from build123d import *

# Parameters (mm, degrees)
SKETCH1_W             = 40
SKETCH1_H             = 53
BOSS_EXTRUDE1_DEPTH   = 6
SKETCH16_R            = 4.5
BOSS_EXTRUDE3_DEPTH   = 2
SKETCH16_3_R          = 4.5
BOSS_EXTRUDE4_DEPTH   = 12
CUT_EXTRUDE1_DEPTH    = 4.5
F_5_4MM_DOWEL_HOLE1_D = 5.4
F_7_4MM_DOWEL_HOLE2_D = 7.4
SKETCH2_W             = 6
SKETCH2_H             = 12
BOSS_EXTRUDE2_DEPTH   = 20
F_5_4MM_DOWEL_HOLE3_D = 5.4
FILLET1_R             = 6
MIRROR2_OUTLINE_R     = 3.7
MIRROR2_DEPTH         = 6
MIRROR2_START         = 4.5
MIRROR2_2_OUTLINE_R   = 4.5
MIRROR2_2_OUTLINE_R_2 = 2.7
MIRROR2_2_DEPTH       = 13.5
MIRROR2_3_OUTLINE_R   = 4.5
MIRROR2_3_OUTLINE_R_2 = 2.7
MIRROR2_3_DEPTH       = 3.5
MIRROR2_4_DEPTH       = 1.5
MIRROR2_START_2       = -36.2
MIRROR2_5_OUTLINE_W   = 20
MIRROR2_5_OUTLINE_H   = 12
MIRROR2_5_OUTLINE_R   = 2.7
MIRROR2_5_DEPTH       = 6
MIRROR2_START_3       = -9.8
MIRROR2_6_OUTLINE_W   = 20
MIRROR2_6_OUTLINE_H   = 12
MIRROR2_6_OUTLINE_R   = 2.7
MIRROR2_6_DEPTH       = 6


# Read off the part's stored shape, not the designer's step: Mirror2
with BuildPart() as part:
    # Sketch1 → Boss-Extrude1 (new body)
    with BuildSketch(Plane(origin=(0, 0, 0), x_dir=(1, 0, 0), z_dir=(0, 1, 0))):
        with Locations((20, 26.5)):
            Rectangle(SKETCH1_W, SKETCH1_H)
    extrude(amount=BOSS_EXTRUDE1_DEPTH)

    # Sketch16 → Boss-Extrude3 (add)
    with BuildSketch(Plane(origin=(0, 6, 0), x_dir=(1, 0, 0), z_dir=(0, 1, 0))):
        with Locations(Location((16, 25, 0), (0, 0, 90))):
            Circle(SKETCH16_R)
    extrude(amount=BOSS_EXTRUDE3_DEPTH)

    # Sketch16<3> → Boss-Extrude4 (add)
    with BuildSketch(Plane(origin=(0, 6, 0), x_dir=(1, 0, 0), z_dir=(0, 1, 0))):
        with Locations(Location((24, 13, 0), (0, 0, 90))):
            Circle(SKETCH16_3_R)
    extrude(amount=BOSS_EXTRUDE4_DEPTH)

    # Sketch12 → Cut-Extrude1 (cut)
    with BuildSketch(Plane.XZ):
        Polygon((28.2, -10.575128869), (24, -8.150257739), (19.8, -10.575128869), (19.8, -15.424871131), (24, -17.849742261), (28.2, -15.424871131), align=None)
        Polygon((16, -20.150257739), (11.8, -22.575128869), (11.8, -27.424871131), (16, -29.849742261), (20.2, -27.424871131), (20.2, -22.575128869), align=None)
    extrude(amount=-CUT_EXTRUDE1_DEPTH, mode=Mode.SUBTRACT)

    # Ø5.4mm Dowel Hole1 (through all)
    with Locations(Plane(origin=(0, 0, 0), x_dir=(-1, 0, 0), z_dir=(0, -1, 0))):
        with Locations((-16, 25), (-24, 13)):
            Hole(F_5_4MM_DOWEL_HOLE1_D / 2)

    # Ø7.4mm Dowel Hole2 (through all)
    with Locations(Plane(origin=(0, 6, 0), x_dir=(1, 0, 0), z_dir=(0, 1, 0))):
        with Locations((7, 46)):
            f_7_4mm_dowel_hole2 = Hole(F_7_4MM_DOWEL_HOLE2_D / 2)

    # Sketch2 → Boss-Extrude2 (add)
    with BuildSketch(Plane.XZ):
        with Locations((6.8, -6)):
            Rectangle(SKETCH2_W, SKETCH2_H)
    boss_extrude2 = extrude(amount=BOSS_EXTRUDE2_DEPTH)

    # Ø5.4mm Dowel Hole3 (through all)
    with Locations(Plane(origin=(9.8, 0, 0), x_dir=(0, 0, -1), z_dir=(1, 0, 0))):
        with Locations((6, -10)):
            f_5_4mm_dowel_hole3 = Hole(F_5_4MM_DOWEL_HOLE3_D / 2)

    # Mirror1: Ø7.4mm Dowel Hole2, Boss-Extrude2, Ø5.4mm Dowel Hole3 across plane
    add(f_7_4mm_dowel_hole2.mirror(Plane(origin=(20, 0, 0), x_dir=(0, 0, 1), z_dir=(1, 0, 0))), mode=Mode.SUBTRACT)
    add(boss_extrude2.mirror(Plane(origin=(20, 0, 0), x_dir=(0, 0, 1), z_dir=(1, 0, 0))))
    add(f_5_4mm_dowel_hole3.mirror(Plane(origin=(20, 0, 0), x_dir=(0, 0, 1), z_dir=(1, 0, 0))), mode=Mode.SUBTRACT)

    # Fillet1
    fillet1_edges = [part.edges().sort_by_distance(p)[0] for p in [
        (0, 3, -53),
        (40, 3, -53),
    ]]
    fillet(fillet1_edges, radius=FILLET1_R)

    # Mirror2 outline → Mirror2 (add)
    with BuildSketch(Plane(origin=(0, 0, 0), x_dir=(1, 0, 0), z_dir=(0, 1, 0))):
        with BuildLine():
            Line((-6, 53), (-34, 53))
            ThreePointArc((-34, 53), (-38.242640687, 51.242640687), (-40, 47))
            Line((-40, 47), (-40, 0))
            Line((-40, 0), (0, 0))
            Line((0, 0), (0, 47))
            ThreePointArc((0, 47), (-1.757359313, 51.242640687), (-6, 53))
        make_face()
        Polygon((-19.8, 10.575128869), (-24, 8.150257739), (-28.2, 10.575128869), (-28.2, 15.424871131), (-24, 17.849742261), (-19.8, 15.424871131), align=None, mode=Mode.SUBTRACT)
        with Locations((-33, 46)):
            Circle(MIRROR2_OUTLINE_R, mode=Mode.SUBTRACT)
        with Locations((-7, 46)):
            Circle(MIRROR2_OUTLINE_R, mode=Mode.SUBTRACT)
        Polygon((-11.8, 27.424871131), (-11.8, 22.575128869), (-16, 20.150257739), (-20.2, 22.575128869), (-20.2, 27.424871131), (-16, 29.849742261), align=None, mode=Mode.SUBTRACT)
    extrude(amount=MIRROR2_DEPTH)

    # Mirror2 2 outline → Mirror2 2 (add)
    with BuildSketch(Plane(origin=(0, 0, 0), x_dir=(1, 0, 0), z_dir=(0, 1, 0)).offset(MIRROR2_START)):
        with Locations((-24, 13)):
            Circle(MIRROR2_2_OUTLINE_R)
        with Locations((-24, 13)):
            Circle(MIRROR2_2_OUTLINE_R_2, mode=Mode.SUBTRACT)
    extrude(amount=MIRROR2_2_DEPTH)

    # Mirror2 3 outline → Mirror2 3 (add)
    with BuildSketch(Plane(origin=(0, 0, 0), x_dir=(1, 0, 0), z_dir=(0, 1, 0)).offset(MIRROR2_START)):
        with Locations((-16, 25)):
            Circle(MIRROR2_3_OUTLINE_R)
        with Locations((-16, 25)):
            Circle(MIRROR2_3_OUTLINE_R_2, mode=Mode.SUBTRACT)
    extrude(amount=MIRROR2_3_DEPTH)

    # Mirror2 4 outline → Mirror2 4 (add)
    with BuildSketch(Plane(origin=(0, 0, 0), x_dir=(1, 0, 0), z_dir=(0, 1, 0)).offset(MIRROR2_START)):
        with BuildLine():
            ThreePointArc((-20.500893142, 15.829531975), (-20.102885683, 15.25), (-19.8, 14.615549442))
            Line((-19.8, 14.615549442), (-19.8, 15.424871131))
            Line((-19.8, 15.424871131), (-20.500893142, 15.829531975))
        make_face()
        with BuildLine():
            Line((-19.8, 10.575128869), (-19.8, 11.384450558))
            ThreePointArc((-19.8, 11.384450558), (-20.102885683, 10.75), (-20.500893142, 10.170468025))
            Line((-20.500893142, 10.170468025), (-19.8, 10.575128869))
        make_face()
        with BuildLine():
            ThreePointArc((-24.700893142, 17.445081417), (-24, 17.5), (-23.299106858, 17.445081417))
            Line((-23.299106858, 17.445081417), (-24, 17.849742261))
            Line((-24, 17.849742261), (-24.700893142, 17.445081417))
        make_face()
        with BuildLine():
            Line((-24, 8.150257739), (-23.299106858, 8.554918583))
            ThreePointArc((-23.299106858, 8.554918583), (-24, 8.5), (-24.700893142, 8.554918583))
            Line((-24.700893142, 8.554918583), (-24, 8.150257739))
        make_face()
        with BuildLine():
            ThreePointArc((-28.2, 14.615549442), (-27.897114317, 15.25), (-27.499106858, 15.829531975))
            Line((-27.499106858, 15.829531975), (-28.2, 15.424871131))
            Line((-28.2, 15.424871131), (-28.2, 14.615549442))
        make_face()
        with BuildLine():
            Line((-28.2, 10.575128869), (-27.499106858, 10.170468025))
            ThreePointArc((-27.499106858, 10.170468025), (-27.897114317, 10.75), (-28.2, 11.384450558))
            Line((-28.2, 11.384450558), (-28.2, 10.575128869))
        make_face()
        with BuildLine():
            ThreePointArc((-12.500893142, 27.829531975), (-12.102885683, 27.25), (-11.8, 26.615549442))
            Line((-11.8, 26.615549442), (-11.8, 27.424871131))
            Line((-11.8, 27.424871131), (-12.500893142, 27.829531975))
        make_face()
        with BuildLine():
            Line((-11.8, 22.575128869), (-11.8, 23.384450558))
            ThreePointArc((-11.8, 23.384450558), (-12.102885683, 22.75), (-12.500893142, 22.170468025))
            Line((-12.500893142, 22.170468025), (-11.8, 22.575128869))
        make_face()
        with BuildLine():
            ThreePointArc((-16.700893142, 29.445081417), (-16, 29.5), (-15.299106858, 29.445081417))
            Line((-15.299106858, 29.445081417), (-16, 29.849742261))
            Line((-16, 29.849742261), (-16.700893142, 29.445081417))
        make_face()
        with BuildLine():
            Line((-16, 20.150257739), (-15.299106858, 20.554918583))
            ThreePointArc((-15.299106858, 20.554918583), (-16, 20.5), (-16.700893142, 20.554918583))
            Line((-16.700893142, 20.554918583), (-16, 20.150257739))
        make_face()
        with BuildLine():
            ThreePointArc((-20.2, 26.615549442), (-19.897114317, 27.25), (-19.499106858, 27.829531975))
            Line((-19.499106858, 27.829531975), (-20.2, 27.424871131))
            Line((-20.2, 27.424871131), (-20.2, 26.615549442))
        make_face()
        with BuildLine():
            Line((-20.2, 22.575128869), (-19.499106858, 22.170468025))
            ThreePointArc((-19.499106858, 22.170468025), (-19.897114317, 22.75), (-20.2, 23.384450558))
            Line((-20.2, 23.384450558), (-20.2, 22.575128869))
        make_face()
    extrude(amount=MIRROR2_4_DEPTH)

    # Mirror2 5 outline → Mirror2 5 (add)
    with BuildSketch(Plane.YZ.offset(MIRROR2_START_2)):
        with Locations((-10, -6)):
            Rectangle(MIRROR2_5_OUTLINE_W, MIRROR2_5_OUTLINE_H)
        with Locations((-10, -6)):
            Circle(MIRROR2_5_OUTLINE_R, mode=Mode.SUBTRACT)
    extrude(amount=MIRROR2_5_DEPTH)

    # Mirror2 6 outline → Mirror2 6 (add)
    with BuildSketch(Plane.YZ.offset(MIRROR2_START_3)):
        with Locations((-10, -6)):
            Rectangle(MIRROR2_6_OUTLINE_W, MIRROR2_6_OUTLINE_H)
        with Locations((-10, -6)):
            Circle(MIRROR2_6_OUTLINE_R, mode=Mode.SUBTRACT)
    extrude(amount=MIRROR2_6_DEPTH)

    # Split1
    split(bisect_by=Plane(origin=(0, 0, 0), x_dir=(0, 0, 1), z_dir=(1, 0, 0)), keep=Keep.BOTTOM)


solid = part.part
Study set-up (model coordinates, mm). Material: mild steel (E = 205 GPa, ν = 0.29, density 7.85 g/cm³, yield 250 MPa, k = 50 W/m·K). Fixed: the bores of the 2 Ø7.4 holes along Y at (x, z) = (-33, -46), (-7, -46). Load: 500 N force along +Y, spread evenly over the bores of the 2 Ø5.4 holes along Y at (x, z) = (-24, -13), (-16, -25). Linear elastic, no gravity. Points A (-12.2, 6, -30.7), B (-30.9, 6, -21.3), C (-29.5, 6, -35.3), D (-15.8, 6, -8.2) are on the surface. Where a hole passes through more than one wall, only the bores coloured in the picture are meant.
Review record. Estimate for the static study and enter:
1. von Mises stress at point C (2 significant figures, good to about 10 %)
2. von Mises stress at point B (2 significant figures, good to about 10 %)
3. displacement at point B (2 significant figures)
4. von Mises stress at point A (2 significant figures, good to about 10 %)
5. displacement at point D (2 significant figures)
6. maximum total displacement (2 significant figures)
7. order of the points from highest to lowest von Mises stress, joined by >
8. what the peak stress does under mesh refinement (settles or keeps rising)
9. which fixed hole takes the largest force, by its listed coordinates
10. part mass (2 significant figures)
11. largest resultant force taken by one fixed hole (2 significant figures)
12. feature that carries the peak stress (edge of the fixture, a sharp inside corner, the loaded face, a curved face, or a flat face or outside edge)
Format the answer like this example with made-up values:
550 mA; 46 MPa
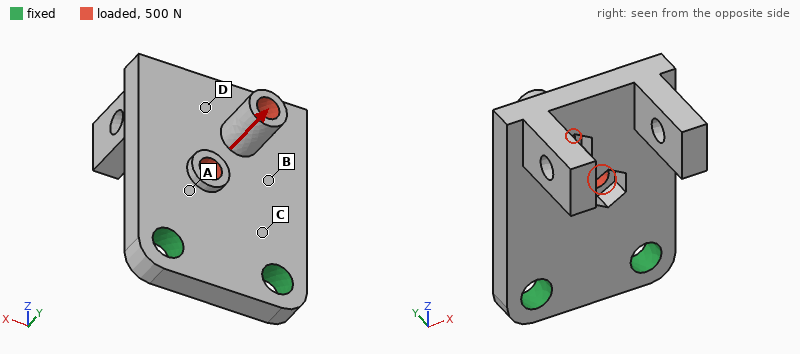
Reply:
41 MPa; 16 MPa; 21 µm; 31 MPa; 40 µm; 66 µm; C > A > B > D; keeps rising; (-33, -46); 120 g; 290 N; edge of the fixture
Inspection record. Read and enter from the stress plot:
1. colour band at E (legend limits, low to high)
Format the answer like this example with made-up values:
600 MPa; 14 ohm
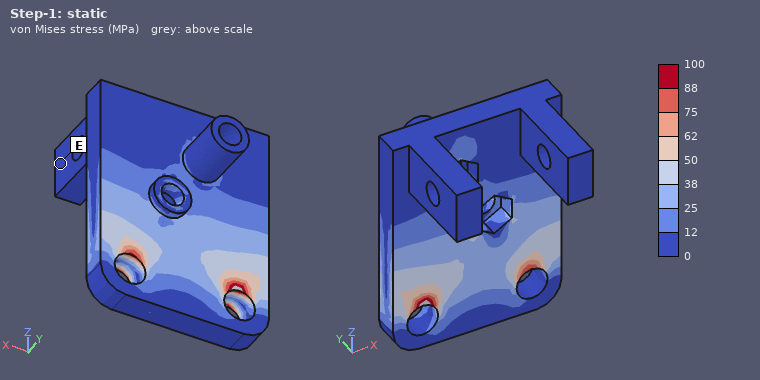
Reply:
0 to 12 MPa
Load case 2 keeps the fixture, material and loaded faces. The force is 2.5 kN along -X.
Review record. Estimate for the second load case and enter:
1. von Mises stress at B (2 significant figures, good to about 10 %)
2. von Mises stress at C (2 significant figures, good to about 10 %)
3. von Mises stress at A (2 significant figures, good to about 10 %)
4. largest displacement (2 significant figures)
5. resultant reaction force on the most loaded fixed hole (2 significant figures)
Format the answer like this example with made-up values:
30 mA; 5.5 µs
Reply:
68 MPa; 65 MPa; 62 MPa; 62 µm; 2.8 kN
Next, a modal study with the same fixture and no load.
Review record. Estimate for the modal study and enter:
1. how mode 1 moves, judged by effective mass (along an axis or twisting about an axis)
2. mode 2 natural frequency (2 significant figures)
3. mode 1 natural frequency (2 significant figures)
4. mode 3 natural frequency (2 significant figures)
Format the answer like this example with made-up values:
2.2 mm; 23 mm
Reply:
along Y; 3700 Hz; 1800 Hz; 6500 Hz
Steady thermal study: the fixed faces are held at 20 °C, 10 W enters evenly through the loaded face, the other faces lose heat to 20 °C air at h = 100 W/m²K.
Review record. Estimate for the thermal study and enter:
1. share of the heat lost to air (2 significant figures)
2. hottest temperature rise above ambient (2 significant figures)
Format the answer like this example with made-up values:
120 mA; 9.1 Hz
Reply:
58 %; 36 K
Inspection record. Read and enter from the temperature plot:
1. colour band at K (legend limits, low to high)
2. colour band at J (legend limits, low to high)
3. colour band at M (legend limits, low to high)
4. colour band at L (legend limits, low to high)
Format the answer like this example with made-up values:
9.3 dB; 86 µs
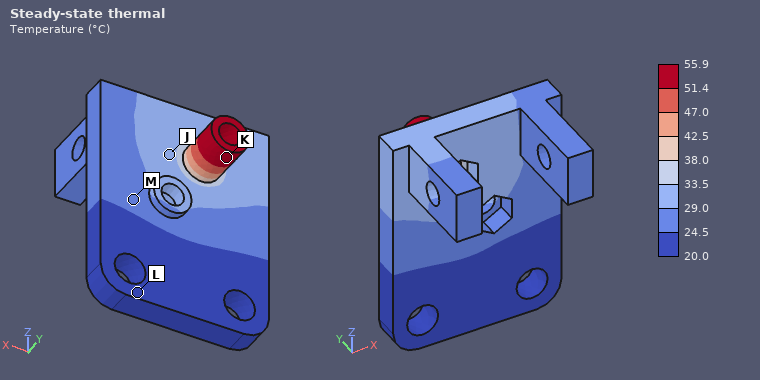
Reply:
51.4 to 55.9 °C; 29.0 to 33.5 °C; 24.5 to 29.0 °C; 20.0 to 24.5 °C
